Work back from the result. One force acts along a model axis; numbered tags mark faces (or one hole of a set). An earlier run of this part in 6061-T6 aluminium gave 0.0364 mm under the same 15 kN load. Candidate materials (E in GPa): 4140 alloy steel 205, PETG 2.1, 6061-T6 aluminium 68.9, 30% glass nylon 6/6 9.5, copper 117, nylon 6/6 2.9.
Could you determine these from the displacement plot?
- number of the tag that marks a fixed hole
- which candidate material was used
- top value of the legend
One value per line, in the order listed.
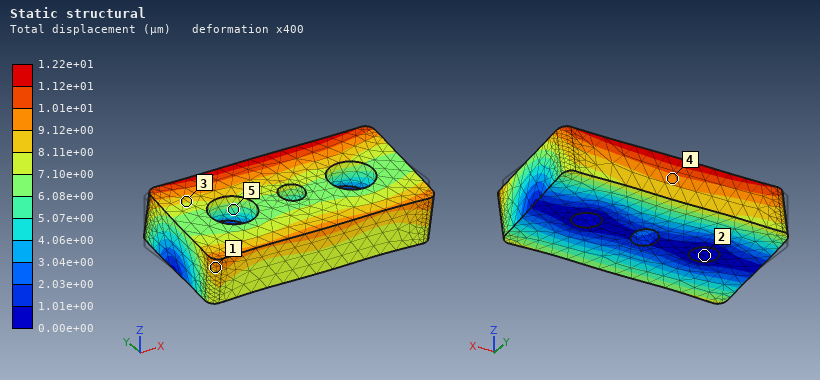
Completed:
2
4140 alloy steel
1.22e+01 µm
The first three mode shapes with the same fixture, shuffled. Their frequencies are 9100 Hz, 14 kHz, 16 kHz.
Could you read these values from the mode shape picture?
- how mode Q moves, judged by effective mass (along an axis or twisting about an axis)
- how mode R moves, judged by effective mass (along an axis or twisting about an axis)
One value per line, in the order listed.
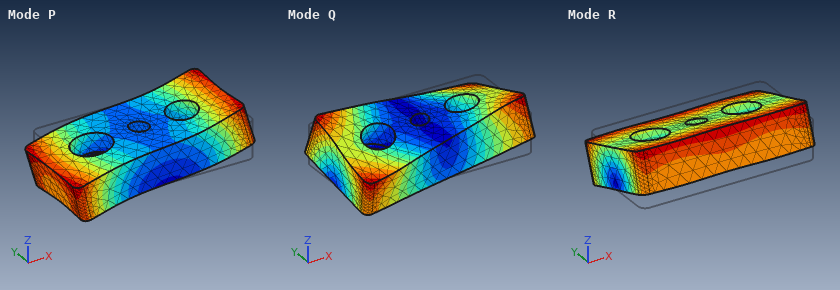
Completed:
twisting about Z
along Y
